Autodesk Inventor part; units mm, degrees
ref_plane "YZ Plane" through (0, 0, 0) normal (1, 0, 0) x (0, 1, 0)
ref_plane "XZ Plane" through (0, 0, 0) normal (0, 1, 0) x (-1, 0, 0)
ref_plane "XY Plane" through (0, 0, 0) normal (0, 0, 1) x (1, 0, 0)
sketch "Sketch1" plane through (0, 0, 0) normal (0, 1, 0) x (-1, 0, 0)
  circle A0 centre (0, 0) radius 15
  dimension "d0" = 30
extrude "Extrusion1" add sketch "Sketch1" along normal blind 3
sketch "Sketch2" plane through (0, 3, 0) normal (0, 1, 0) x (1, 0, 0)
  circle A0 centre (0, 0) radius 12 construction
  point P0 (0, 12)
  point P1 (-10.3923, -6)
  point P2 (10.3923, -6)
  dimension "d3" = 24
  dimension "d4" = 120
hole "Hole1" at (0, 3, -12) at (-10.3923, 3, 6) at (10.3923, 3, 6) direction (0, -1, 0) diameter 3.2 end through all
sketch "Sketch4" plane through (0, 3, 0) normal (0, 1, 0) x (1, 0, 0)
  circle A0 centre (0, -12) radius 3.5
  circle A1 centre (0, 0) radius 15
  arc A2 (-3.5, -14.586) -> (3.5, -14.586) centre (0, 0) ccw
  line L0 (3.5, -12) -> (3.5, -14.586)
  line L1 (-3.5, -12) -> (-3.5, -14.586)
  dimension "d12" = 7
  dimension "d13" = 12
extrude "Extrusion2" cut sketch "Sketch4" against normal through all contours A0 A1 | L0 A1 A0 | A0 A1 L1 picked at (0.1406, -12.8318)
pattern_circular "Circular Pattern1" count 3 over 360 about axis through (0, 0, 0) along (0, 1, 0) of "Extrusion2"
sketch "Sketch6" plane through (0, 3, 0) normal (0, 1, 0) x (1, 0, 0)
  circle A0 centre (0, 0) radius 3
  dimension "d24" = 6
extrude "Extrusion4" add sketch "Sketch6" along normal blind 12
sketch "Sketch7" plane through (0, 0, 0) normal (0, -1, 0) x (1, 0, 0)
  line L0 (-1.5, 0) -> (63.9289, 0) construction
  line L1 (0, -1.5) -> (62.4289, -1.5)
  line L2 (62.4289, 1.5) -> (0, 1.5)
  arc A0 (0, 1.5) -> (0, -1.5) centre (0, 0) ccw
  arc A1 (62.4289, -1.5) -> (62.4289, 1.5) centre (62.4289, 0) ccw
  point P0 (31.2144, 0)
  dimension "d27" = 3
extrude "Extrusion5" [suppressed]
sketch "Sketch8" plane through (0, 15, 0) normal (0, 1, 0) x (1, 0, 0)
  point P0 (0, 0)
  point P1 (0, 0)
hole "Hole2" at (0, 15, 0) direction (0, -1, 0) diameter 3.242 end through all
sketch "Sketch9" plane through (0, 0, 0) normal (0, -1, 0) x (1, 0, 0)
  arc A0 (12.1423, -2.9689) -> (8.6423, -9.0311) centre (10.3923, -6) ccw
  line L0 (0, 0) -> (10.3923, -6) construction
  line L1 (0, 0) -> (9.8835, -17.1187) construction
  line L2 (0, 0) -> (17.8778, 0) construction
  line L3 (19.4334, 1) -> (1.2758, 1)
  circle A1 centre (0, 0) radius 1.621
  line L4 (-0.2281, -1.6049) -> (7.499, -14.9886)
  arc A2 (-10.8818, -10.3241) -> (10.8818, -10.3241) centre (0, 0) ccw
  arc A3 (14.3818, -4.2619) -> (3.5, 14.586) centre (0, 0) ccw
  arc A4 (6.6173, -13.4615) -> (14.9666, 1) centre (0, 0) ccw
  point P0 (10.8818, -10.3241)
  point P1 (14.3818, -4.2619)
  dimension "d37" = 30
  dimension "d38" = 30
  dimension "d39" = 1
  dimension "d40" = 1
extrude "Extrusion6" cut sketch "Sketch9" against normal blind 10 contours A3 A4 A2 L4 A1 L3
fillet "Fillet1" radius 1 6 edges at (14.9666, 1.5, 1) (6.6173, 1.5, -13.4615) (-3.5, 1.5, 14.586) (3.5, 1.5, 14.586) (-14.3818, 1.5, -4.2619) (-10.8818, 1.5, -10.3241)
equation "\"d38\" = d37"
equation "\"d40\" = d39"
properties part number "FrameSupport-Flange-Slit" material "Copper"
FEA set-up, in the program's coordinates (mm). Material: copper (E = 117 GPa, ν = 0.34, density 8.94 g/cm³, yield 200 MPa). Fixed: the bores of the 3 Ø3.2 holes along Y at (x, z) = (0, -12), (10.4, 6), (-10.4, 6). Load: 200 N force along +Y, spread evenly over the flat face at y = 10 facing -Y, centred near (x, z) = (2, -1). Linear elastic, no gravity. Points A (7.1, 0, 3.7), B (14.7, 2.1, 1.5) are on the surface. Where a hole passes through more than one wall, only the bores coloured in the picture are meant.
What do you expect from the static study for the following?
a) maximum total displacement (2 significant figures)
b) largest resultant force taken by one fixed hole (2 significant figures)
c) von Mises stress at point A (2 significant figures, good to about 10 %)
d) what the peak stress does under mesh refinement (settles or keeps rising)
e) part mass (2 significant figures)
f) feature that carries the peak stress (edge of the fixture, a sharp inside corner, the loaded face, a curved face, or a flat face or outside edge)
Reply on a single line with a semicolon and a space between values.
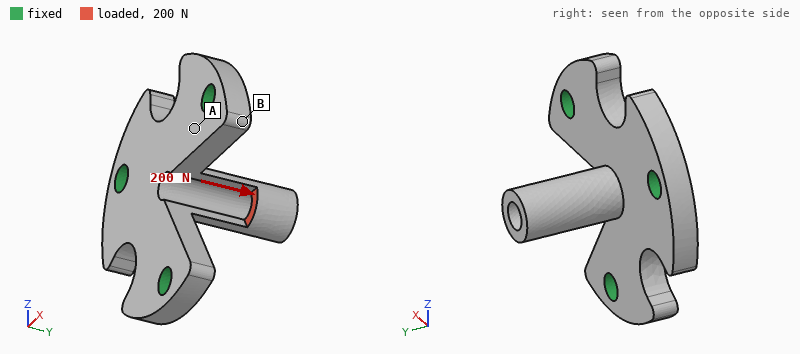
30 µm; 82 N; 20 MPa; keeps rising; 14 g; a sharp inside corner
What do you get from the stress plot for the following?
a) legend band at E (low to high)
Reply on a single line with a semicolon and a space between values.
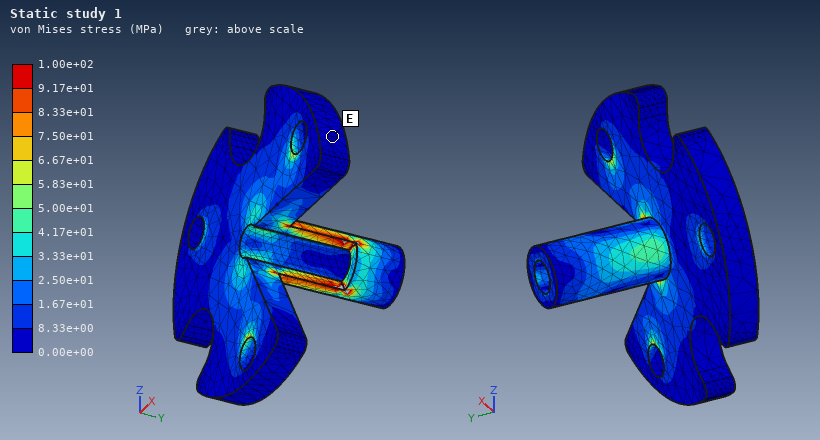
0.00e+00 to 8.33e+00 MPa
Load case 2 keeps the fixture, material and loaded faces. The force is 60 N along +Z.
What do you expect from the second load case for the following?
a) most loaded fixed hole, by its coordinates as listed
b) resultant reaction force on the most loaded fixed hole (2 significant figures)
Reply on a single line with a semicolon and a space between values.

(0, -12); 40 N
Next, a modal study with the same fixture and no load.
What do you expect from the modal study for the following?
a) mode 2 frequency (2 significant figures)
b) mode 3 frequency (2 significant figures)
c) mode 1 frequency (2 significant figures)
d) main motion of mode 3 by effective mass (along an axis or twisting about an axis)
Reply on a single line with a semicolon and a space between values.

9900 Hz; 20 kHz; 9700 Hz; along Y
